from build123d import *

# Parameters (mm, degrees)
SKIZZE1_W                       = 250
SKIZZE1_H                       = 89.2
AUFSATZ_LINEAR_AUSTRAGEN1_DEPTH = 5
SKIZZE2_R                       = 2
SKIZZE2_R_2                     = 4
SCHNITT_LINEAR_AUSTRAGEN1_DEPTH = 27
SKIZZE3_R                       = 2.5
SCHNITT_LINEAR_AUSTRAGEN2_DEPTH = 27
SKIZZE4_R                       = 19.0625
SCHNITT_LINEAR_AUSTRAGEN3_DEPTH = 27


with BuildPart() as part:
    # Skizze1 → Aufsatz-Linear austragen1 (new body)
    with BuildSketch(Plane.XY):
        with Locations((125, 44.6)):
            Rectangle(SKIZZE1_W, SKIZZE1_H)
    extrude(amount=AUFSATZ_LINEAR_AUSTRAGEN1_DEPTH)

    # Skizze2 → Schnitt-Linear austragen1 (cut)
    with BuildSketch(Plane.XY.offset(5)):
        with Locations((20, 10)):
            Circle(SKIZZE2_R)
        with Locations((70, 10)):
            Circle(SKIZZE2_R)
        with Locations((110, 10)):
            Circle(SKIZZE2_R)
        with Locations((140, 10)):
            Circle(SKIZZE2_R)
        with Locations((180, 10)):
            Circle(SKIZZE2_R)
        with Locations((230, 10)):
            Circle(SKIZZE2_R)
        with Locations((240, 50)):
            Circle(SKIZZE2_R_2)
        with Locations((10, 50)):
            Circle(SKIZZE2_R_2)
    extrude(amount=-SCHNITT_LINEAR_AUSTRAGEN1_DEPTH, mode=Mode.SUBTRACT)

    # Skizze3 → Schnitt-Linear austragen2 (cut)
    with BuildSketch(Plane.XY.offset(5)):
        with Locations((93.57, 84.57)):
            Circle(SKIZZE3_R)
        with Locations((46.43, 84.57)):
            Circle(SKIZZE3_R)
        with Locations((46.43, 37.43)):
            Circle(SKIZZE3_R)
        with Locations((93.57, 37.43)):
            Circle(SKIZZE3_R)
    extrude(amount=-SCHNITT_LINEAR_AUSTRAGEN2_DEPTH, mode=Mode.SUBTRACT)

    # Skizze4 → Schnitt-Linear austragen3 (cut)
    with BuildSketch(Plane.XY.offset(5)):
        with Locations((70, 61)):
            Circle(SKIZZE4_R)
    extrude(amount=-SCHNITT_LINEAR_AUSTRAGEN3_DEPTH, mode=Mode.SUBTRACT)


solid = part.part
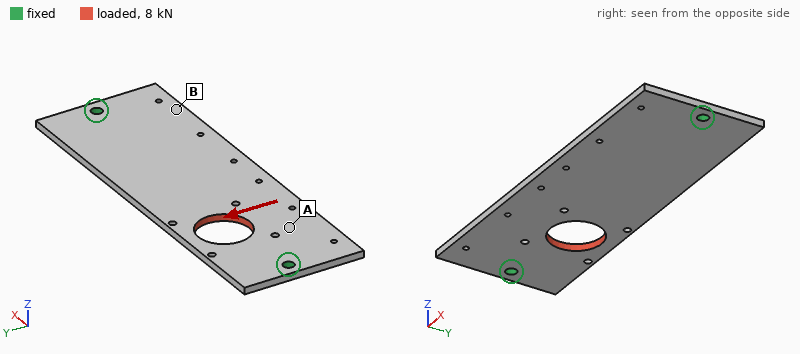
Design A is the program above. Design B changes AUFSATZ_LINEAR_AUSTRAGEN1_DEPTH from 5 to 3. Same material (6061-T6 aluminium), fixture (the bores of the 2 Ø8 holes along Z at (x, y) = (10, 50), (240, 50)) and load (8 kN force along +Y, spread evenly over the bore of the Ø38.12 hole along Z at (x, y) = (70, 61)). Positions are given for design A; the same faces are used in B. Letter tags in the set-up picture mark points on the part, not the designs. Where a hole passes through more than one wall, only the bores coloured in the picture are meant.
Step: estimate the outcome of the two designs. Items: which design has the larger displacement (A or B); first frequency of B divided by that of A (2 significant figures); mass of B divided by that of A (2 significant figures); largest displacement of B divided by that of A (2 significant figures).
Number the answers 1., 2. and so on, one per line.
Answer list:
1. B
2. 0.61
3. 0.60
4. 1.7
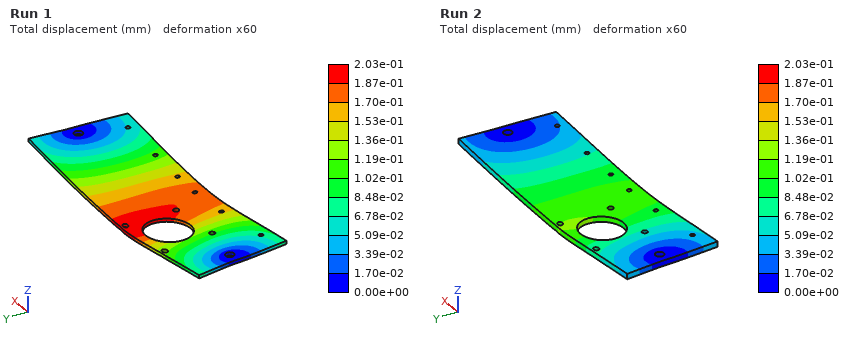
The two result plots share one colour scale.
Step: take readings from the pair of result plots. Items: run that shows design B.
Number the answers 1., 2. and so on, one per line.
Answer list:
1. Run 1
